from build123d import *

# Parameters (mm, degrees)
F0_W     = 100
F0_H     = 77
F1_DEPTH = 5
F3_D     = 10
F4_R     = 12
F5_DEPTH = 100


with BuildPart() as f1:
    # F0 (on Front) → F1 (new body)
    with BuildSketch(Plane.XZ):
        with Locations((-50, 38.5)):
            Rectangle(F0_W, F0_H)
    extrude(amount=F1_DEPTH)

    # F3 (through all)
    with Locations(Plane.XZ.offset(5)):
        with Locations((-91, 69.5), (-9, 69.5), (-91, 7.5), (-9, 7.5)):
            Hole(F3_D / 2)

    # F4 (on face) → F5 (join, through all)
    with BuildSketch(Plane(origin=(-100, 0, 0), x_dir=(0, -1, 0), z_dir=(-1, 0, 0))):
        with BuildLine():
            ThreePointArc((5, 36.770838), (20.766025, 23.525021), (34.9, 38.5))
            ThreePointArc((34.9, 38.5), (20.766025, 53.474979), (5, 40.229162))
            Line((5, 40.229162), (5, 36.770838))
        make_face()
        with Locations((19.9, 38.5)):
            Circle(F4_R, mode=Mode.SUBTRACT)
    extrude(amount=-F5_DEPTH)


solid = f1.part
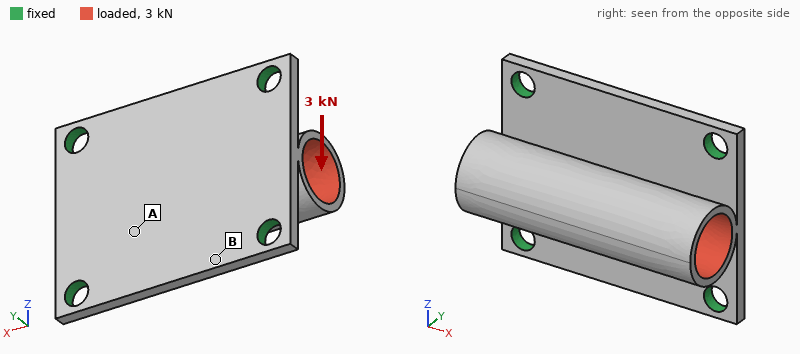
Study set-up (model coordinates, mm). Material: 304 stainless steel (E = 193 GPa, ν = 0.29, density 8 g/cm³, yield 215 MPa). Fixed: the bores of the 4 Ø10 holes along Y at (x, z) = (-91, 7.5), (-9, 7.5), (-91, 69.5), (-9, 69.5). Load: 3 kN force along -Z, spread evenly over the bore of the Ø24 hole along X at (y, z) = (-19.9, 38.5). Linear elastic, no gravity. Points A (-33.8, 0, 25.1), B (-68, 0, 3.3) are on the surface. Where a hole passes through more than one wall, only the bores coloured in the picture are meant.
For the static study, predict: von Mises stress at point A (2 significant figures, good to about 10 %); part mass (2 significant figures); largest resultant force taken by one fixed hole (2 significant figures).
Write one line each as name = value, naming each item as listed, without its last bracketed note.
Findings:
von Mises stress at point A = 25 MPa
part mass = 500 g
largest resultant force taken by one fixed hole = 990 N
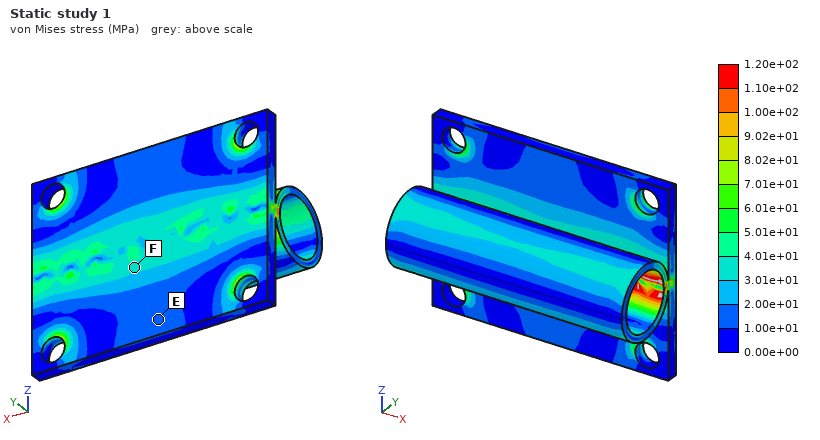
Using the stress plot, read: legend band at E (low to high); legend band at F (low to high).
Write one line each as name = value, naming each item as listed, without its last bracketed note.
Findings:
legend band at E = 1.00e+01 to 2.00e+01 MPa
legend band at F = 3.01e+01 to 4.01e+01 MPa
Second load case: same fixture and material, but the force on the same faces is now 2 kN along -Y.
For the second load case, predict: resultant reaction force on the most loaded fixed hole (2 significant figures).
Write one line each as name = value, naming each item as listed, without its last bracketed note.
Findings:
resultant reaction force on the most loaded fixed hole = 500 N
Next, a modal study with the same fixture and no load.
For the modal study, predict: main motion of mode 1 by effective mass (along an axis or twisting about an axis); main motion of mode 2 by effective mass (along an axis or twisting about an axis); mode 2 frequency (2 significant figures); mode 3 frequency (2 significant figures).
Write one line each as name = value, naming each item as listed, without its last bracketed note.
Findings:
main motion of mode 1 by effective mass = along Z
main motion of mode 2 by effective mass = along Y
mode 2 frequency = 2900 Hz
mode 3 frequency = 3400 Hz
